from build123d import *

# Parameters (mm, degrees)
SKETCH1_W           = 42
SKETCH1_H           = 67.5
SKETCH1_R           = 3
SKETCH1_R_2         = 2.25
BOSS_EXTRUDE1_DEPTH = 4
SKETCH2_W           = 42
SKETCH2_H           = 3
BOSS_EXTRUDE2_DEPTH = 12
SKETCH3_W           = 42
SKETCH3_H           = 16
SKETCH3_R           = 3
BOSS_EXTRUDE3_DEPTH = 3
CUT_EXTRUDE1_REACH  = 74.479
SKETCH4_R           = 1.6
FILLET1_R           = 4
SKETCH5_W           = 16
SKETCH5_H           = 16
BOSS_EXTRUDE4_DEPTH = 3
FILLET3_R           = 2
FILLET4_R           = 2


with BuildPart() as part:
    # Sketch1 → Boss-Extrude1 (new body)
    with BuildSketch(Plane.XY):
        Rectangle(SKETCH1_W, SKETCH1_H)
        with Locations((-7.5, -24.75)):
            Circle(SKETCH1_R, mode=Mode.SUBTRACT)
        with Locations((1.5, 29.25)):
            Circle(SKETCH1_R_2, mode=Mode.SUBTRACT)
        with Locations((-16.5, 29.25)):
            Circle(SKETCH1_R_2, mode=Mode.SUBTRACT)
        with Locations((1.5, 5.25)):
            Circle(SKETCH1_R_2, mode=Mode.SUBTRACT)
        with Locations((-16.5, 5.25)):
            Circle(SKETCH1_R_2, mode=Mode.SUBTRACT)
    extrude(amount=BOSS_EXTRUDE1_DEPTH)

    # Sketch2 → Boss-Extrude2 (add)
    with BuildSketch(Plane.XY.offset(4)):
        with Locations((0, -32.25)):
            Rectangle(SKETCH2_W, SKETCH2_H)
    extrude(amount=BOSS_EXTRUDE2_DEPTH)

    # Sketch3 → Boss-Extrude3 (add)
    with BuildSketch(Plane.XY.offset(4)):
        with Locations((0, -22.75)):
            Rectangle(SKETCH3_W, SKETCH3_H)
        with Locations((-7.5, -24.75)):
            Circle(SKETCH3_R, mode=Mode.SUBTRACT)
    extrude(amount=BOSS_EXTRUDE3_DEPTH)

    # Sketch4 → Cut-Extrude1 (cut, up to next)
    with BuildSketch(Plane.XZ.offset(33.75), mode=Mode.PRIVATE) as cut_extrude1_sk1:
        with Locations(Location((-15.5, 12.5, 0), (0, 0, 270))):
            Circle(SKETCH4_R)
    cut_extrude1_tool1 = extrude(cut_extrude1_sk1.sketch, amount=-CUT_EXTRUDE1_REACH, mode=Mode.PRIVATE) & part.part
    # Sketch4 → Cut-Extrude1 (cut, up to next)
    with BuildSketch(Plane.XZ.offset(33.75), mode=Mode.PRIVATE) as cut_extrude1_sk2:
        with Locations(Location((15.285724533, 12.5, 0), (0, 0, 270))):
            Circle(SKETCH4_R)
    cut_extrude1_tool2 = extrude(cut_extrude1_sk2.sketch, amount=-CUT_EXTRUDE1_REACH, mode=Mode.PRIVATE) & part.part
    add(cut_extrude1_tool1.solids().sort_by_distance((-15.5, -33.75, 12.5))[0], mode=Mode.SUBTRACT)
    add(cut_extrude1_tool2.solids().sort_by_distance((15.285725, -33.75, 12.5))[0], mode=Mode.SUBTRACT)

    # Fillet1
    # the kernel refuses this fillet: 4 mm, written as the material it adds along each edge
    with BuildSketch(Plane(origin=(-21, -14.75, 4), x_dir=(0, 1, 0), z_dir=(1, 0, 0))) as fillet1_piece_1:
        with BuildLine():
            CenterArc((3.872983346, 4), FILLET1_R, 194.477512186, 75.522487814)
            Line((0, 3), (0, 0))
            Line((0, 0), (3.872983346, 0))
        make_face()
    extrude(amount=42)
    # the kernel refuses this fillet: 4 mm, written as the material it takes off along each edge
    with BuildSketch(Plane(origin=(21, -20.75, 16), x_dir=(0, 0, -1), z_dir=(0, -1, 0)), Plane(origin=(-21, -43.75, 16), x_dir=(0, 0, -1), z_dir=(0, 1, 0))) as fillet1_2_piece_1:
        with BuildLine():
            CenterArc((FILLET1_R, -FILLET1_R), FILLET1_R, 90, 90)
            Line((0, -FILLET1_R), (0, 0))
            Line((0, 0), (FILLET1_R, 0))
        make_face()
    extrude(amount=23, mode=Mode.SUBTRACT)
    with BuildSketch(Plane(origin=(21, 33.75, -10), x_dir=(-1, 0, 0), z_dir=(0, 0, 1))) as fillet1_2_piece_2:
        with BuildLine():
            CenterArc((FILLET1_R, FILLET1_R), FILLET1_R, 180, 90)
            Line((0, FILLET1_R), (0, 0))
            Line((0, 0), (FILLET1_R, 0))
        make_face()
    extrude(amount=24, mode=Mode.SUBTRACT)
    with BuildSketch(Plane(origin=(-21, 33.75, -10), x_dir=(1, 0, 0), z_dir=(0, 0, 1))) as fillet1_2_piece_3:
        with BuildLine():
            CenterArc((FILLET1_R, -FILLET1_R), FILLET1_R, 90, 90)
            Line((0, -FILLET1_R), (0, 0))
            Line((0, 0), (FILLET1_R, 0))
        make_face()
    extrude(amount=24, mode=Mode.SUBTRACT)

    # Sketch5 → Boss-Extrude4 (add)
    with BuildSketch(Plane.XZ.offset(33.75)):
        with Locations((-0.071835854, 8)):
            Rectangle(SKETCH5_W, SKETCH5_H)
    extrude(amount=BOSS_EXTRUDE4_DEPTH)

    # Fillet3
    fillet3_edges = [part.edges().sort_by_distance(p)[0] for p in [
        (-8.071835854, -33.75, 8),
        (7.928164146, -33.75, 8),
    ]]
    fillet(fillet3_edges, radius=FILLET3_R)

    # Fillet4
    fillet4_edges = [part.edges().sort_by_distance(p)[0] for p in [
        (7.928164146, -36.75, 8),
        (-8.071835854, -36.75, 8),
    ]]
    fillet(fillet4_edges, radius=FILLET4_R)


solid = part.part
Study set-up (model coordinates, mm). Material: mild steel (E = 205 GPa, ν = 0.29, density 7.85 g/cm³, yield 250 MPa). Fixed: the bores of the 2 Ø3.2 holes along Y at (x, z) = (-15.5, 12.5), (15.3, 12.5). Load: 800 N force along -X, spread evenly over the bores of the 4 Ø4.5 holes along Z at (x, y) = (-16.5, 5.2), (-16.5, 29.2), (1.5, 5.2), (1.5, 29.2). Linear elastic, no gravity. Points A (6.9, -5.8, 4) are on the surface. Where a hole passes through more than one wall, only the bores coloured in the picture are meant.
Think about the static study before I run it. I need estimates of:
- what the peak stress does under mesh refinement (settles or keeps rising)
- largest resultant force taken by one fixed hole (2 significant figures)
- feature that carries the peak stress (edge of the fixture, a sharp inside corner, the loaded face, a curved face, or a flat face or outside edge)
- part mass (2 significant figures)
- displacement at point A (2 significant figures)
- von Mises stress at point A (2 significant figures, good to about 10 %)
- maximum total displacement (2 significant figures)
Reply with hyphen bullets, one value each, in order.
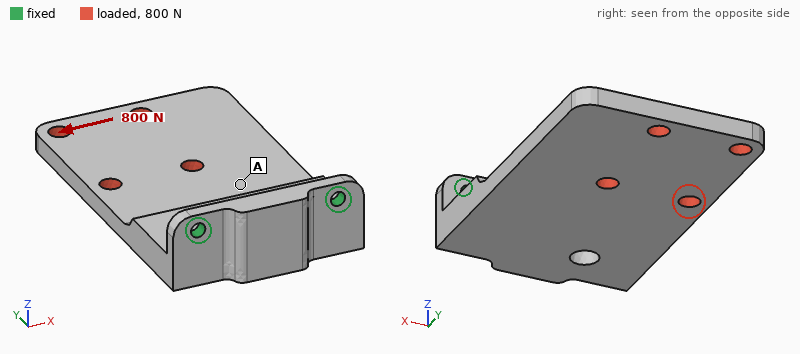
- keeps rising
- 1.4 kN
- edge of the fixture
- 120 g
- 24 µm
- 18 MPa
- 63 µm
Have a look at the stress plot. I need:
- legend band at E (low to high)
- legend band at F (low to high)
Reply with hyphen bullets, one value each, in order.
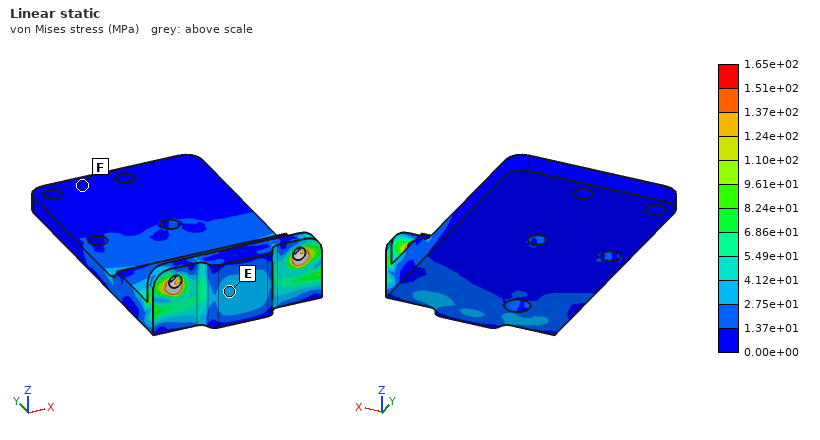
- 2.75e+01 to 4.12e+01 MPa
- 0.00e+00 to 1.37e+01 MPa
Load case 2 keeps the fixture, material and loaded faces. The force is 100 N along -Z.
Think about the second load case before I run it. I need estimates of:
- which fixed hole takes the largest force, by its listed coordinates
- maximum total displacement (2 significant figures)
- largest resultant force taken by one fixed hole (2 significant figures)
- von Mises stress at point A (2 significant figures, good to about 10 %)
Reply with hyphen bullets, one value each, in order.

- (-15.5, 12.5)
- 0.18 mm
- 76 N
- 19 MPa
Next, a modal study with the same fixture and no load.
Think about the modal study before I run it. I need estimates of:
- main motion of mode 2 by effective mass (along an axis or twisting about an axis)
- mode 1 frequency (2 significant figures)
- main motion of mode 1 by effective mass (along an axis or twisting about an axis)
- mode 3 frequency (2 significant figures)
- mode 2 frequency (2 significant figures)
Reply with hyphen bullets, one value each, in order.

- along X
- 660 Hz
- along Z
- 3400 Hz
- 2700 Hz
